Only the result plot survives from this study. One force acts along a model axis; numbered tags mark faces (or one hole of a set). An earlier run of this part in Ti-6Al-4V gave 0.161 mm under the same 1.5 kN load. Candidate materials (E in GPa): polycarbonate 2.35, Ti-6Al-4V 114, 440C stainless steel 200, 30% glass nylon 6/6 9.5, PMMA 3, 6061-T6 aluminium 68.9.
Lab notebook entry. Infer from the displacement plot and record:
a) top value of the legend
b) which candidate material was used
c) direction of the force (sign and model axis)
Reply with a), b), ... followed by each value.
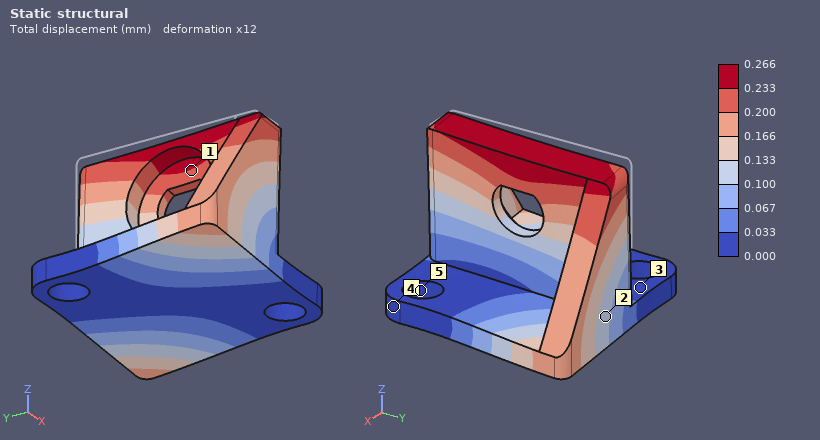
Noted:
a) 0.266 mm
b) 6061-T6 aluminium
c) +X
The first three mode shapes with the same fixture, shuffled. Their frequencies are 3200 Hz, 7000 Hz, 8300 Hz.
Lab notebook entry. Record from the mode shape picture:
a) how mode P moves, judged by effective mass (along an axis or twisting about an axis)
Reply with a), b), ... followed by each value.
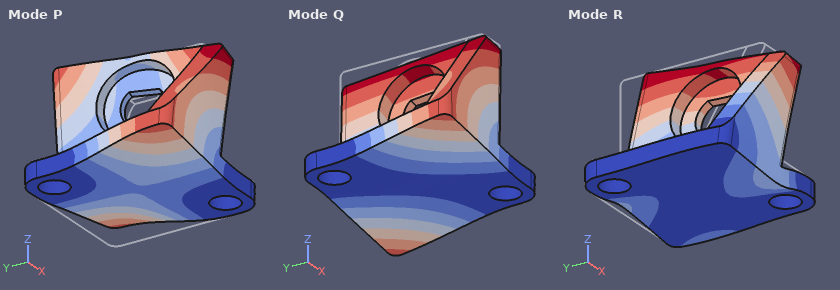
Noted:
a) along Z
